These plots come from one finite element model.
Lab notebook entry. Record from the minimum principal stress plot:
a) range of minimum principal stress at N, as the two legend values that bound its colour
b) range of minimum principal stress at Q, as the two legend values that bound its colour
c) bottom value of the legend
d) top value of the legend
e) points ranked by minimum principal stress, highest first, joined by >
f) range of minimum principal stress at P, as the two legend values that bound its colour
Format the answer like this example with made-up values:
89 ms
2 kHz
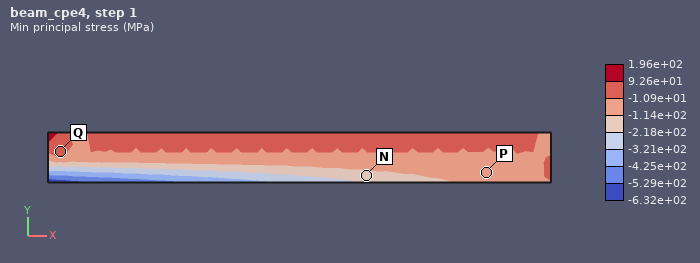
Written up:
-2.18e+02 to -1.14e+02 MPa
-1.09e+01 to 9.26e+01 MPa
-6.32e+02 MPa
1.96e+02 MPa
Q > P > N
-1.14e+02 to -1.09e+01 MPa
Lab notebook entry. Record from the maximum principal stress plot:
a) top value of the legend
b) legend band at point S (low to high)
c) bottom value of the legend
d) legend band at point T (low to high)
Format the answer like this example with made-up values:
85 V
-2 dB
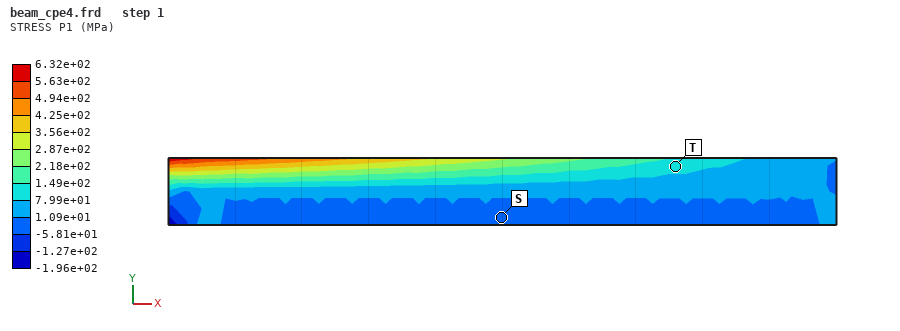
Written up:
6.32e+02 MPa
-5.81e+01 to 1.09e+01 MPa
-1.96e+02 MPa
7.99e+01 to 1.49e+02 MPa
